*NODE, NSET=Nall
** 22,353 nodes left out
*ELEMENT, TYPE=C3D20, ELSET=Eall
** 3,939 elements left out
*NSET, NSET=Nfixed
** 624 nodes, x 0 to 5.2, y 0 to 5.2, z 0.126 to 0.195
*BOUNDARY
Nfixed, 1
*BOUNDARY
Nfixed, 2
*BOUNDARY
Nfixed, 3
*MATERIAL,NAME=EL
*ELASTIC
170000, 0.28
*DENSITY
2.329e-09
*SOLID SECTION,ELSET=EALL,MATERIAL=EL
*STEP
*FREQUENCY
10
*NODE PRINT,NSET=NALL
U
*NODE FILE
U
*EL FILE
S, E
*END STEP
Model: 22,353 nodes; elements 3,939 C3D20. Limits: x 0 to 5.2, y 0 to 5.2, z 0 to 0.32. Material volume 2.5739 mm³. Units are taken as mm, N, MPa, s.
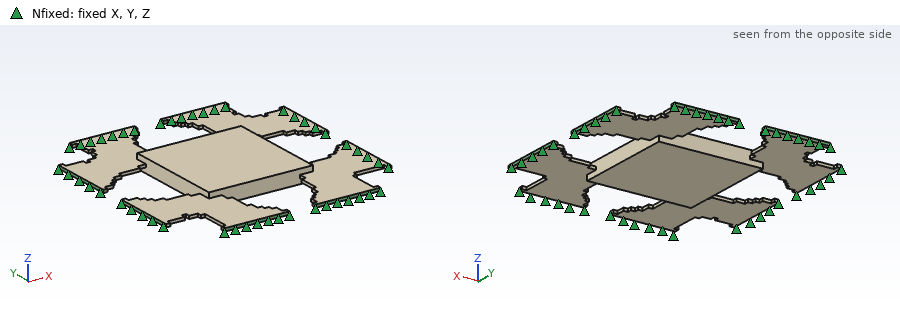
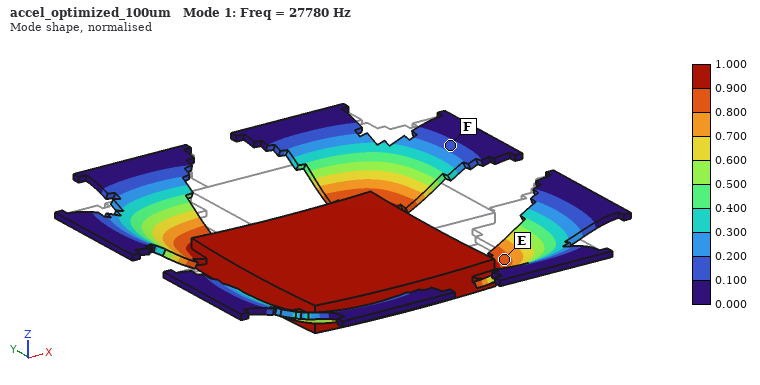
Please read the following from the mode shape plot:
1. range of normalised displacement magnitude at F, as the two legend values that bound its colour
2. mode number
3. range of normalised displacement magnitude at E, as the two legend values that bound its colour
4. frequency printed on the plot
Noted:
0.100 to 0.200
1
0.800 to 0.900
27780 Hz
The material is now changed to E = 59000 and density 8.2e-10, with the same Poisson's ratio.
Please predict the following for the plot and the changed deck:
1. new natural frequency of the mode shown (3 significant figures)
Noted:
27600 Hz
